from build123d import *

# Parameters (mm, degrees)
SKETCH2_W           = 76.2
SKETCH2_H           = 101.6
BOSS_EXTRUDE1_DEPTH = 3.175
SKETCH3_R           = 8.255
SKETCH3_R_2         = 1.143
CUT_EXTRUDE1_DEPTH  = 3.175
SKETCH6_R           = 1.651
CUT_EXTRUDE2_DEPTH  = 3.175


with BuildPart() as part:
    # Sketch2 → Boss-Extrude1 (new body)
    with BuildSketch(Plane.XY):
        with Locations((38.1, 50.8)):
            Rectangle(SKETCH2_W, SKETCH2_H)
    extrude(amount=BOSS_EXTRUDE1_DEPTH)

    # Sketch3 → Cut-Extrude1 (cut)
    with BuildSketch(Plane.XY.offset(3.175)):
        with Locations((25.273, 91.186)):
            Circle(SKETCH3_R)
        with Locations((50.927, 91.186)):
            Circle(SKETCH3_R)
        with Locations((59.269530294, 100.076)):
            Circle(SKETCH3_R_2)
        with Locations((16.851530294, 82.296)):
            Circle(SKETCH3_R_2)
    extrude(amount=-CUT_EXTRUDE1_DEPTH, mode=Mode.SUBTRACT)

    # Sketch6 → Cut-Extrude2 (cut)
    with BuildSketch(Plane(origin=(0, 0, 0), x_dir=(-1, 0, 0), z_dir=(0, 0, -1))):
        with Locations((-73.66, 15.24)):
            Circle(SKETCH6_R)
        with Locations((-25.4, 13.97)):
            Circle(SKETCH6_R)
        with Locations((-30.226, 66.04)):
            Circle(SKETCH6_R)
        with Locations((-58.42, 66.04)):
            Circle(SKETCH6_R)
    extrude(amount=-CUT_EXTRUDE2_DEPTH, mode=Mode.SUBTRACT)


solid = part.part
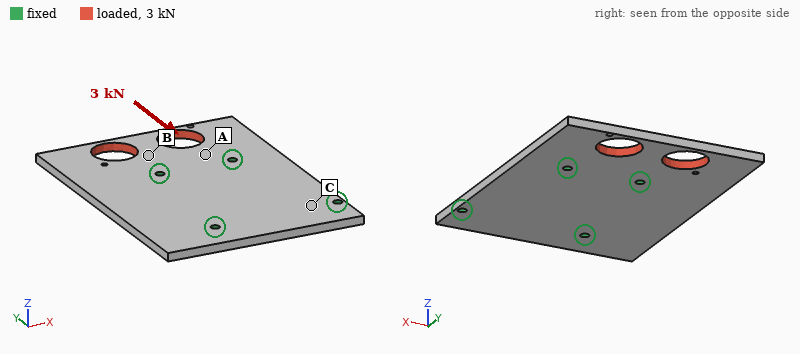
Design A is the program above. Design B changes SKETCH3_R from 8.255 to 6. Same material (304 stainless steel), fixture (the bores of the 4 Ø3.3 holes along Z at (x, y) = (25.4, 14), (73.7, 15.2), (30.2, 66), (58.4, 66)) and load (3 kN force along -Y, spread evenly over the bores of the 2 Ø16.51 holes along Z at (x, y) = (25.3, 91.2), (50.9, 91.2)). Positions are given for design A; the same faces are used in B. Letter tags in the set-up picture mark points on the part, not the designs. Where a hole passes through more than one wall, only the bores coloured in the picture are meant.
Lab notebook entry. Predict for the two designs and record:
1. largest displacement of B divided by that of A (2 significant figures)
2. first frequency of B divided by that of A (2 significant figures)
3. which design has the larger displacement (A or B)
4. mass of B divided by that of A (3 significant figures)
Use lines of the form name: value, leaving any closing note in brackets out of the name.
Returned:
largest displacement of B divided by that of A: 0.66
first frequency of B divided by that of A: 0.99
which design has the larger displacement: A
mass of B divided by that of A: 1.03
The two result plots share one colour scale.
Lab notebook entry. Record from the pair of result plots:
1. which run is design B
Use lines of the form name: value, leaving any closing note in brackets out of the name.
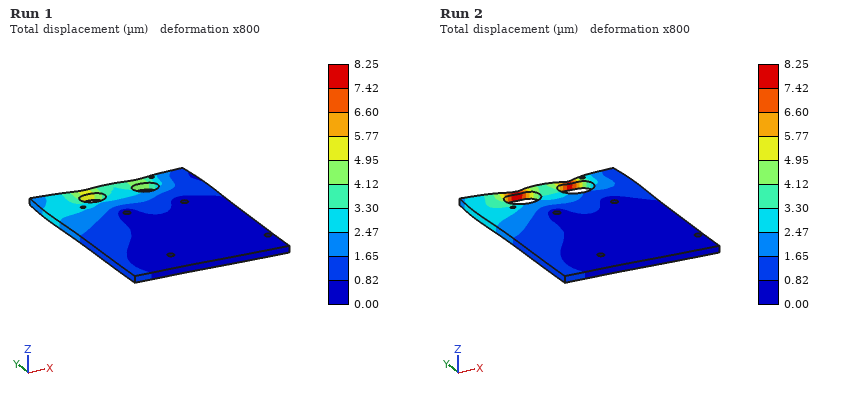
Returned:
which run is design B: Run 1
